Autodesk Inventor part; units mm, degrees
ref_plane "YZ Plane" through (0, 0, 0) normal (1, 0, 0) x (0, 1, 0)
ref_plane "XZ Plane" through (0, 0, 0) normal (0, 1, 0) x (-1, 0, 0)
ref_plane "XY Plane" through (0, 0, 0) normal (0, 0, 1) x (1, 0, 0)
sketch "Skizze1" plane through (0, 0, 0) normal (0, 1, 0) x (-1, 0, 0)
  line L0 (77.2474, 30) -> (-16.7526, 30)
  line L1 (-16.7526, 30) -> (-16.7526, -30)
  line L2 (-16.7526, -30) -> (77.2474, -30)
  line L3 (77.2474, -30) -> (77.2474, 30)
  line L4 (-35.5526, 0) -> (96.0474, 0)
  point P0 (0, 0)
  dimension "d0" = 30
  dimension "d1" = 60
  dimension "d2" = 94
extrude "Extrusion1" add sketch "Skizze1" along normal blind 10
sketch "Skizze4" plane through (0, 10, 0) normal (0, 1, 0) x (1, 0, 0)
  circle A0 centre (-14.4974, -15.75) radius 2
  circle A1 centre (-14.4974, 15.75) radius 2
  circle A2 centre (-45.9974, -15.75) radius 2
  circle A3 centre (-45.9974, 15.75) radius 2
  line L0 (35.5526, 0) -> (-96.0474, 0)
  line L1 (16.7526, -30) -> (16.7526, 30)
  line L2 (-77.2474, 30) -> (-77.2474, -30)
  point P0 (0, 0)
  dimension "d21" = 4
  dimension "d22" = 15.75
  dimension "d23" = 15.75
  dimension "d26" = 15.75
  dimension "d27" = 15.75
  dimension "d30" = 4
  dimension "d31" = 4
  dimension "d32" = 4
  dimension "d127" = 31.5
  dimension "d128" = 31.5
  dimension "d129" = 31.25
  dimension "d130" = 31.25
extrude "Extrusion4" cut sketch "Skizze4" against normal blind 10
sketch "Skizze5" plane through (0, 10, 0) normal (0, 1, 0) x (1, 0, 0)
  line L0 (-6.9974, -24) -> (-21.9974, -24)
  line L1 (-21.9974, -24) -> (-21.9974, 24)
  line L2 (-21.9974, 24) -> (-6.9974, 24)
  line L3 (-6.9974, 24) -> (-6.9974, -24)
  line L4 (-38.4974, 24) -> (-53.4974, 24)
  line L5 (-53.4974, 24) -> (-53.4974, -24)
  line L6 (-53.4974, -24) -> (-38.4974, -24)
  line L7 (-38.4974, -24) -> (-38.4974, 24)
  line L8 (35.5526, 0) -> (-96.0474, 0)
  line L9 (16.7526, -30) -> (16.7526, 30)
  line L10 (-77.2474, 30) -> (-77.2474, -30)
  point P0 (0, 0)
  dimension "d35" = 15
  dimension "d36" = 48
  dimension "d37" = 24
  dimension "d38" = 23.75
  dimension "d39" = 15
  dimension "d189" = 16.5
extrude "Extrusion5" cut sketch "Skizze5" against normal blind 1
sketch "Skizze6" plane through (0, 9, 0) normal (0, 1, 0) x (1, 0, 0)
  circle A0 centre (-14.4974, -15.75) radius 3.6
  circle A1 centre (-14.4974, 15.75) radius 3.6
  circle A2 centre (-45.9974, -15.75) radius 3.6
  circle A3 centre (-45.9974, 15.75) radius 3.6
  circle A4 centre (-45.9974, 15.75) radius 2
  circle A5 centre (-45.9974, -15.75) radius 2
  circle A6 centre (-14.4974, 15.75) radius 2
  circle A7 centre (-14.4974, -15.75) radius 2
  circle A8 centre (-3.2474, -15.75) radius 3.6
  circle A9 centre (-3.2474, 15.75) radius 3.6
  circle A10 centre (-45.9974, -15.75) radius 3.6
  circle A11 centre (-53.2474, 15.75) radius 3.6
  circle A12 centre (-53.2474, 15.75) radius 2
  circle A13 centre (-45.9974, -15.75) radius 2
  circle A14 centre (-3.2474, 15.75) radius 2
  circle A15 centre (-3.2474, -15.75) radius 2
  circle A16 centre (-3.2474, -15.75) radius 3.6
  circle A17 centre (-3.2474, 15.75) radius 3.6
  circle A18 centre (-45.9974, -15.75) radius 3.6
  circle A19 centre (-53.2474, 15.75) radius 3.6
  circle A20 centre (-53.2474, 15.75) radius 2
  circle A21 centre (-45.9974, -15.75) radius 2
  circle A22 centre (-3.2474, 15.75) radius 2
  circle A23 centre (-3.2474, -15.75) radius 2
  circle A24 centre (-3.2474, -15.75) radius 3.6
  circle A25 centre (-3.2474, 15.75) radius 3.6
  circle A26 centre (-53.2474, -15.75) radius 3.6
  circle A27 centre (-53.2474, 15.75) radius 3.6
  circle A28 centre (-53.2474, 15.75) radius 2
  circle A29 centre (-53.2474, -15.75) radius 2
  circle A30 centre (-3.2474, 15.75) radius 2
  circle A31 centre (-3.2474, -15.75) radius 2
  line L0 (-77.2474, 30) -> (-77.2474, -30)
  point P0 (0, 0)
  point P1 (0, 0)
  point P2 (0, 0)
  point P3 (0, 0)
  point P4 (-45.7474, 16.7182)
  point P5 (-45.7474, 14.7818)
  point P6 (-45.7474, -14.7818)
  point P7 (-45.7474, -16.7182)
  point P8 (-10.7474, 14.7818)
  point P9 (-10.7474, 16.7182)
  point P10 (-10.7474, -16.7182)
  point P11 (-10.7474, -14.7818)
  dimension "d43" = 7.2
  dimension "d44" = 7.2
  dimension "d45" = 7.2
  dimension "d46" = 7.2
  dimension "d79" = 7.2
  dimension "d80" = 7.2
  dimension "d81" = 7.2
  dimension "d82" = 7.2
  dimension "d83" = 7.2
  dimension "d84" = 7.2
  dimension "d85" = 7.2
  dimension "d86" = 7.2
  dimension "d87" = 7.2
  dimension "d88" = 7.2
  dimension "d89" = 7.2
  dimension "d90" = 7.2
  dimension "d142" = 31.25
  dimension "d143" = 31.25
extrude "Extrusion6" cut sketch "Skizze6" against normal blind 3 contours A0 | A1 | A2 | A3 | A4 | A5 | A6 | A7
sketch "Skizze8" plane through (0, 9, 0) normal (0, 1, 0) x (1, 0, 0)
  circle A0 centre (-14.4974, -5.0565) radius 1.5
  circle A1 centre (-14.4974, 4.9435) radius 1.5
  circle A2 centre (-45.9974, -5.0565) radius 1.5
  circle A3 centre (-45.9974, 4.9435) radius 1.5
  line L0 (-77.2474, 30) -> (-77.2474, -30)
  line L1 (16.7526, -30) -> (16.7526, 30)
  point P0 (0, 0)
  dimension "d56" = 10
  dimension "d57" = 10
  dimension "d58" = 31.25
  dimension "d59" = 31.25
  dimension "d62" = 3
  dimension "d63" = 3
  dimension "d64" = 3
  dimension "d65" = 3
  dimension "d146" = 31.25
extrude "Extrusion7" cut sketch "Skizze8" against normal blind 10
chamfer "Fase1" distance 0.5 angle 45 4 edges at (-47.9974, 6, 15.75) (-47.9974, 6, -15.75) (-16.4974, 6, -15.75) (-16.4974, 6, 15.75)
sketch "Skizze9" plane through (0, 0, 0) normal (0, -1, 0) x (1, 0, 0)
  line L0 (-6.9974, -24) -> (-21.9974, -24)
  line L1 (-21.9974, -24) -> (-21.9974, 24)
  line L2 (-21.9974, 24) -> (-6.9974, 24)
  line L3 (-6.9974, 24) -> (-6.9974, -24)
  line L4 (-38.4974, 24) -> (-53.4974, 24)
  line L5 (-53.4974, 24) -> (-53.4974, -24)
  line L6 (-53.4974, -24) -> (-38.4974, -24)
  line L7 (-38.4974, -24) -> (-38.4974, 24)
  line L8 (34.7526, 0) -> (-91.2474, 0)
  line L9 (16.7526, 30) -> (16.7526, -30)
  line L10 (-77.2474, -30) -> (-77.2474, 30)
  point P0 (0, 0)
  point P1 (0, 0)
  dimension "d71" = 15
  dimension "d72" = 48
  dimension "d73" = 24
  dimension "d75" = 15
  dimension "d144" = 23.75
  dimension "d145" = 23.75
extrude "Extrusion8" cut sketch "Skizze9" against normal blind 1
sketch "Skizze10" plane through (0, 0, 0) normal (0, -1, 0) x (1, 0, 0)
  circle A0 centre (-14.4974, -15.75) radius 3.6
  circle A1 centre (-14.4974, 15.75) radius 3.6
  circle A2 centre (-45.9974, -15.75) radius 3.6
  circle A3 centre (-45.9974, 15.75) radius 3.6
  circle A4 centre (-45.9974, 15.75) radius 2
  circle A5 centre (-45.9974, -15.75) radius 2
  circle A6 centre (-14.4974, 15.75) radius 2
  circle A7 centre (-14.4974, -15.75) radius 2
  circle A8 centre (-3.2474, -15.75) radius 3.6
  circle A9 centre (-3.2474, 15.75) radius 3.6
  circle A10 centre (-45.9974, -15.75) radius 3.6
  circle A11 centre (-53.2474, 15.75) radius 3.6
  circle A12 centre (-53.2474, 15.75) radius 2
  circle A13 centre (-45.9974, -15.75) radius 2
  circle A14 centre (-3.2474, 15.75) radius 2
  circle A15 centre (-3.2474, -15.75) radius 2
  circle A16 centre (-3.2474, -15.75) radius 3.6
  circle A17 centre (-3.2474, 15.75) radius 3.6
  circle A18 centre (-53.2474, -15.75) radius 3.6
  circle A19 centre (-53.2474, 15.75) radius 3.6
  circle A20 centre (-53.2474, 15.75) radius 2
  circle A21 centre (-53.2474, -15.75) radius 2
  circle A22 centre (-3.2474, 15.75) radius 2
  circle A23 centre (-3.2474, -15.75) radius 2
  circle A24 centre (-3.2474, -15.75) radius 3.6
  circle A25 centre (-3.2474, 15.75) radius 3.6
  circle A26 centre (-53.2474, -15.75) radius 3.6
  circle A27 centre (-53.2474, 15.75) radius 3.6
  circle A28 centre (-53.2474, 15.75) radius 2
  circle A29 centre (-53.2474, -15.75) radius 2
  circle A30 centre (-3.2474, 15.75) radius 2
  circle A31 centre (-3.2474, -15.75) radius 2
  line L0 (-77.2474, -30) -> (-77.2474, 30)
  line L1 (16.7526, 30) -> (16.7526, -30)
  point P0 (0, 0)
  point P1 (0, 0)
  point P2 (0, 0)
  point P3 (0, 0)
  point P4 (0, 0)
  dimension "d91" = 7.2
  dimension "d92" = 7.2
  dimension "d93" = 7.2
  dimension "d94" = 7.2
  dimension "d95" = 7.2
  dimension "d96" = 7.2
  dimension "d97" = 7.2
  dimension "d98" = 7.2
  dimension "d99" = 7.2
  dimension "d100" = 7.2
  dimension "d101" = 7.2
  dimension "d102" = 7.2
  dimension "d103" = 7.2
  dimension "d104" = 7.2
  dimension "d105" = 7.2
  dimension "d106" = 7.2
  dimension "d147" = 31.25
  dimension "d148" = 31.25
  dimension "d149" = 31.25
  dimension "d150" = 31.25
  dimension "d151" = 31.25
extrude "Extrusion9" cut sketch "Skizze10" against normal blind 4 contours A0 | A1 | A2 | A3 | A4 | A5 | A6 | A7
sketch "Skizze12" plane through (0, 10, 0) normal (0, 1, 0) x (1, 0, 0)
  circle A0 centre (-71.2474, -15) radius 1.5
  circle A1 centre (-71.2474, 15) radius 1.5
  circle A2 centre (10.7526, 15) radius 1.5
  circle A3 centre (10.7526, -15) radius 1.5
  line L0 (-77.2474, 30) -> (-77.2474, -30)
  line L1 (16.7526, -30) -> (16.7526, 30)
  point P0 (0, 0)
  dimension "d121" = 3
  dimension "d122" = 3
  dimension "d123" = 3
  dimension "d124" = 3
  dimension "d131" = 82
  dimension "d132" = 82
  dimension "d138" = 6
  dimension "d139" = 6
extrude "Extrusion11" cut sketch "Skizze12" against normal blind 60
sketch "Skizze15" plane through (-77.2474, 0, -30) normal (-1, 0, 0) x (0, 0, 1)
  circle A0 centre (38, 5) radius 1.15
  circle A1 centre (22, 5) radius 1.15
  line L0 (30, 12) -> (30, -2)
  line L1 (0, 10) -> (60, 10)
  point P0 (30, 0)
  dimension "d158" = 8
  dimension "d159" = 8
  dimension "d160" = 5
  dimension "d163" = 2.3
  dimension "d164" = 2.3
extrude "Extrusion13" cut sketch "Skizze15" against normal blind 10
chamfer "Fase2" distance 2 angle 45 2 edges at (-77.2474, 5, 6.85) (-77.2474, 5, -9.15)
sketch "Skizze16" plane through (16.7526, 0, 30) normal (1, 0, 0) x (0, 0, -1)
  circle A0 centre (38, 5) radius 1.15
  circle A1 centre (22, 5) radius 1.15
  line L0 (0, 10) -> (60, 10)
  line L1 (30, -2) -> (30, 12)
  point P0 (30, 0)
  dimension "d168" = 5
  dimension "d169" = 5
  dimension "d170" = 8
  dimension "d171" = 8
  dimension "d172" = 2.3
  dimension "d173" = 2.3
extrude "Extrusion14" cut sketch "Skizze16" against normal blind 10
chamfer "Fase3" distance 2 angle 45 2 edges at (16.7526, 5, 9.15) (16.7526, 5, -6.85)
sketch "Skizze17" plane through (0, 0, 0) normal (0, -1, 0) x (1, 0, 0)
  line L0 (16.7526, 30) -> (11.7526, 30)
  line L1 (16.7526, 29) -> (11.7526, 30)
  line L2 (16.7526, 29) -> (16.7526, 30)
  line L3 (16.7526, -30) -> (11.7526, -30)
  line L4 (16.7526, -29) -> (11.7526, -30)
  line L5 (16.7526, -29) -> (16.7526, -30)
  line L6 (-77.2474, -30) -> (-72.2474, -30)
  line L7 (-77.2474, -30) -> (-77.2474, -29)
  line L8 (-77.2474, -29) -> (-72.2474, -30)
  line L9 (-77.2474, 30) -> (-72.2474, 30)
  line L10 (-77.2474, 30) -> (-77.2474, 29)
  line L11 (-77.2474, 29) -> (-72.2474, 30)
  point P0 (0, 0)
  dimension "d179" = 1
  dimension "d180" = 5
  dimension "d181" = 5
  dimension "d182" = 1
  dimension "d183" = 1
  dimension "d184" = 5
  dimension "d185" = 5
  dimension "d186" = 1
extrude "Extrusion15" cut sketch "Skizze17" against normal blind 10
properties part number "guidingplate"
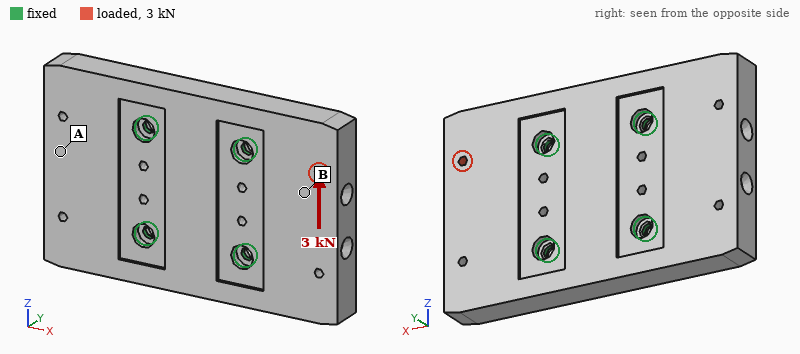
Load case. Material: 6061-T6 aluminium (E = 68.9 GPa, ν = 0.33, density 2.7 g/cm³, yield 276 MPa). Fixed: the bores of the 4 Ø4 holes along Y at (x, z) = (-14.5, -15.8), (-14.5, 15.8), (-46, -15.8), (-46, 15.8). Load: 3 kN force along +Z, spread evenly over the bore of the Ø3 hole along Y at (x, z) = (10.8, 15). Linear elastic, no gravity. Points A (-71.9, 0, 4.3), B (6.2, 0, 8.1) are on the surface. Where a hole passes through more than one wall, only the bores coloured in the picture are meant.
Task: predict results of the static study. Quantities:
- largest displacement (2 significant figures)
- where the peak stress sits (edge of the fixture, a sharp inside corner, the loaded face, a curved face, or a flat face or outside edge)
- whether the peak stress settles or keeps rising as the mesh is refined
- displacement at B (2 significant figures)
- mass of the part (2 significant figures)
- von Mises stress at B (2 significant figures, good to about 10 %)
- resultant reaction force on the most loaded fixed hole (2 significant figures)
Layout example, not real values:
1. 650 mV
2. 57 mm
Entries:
1. 22 µm
2. edge of the fixture
3. keeps rising
4. 13 µm
5. 140 g
6. 18 MPa
7. 2.1 kN
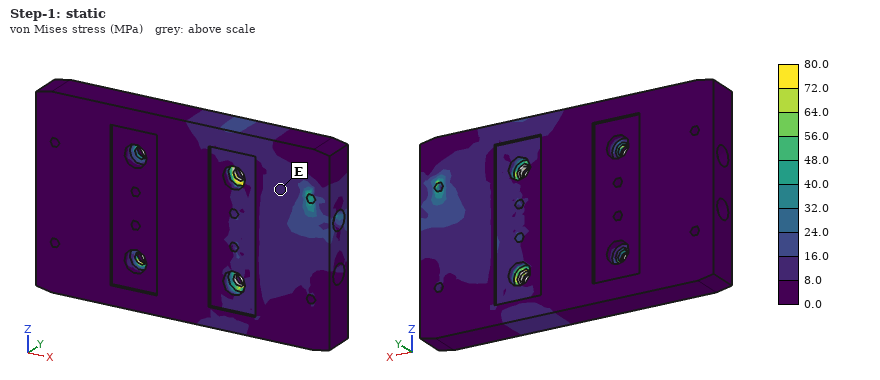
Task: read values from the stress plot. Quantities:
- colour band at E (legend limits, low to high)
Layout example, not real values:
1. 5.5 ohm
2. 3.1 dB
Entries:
1. 8.0 to 16.0 MPa
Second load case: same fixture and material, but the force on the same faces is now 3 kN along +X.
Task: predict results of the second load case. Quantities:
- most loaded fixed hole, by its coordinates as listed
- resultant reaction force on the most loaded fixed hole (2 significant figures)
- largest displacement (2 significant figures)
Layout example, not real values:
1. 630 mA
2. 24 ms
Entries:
1. (-14.5, 15.8)
2. 1.8 kN
3. 11 µm
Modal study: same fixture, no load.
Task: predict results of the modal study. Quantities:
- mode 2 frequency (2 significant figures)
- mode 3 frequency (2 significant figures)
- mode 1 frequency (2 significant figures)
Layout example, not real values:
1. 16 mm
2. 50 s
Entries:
1. 4000 Hz
2. 6900 Hz
3. 3900 Hz
